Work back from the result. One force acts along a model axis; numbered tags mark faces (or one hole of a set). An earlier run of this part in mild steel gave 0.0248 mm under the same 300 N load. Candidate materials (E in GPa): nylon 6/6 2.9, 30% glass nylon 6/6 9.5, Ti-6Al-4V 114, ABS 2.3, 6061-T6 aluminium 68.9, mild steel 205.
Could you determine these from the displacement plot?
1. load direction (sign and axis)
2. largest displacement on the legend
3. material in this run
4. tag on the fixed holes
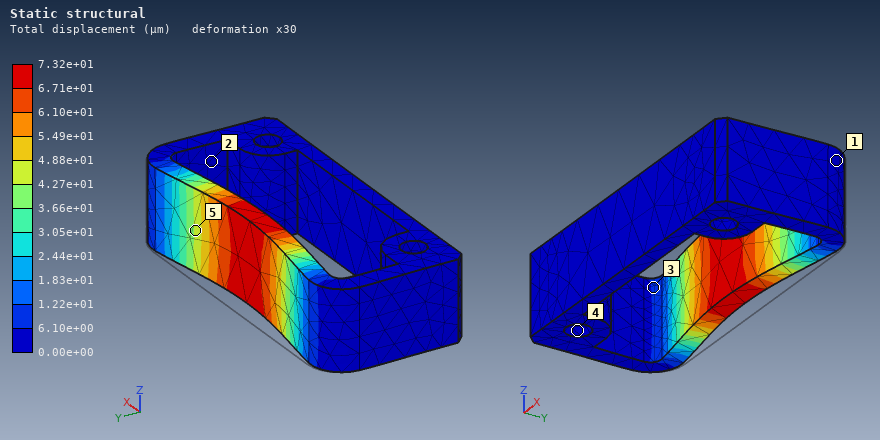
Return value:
-Y
7.32e+01 µm
6061-T6 aluminium
4
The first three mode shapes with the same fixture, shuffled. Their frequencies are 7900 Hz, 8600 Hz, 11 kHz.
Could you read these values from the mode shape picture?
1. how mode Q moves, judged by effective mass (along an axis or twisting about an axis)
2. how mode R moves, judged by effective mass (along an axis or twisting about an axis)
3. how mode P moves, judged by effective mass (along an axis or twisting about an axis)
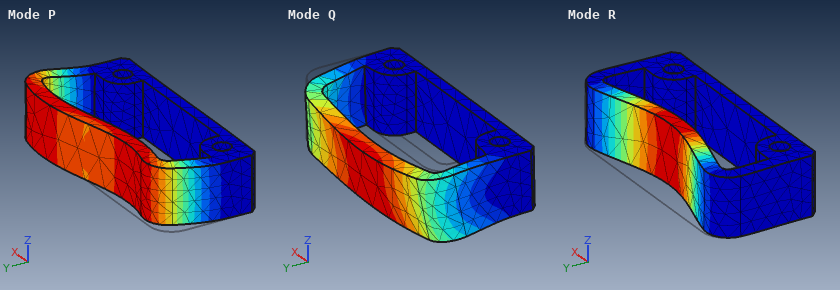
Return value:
along Z
along Y
along X
